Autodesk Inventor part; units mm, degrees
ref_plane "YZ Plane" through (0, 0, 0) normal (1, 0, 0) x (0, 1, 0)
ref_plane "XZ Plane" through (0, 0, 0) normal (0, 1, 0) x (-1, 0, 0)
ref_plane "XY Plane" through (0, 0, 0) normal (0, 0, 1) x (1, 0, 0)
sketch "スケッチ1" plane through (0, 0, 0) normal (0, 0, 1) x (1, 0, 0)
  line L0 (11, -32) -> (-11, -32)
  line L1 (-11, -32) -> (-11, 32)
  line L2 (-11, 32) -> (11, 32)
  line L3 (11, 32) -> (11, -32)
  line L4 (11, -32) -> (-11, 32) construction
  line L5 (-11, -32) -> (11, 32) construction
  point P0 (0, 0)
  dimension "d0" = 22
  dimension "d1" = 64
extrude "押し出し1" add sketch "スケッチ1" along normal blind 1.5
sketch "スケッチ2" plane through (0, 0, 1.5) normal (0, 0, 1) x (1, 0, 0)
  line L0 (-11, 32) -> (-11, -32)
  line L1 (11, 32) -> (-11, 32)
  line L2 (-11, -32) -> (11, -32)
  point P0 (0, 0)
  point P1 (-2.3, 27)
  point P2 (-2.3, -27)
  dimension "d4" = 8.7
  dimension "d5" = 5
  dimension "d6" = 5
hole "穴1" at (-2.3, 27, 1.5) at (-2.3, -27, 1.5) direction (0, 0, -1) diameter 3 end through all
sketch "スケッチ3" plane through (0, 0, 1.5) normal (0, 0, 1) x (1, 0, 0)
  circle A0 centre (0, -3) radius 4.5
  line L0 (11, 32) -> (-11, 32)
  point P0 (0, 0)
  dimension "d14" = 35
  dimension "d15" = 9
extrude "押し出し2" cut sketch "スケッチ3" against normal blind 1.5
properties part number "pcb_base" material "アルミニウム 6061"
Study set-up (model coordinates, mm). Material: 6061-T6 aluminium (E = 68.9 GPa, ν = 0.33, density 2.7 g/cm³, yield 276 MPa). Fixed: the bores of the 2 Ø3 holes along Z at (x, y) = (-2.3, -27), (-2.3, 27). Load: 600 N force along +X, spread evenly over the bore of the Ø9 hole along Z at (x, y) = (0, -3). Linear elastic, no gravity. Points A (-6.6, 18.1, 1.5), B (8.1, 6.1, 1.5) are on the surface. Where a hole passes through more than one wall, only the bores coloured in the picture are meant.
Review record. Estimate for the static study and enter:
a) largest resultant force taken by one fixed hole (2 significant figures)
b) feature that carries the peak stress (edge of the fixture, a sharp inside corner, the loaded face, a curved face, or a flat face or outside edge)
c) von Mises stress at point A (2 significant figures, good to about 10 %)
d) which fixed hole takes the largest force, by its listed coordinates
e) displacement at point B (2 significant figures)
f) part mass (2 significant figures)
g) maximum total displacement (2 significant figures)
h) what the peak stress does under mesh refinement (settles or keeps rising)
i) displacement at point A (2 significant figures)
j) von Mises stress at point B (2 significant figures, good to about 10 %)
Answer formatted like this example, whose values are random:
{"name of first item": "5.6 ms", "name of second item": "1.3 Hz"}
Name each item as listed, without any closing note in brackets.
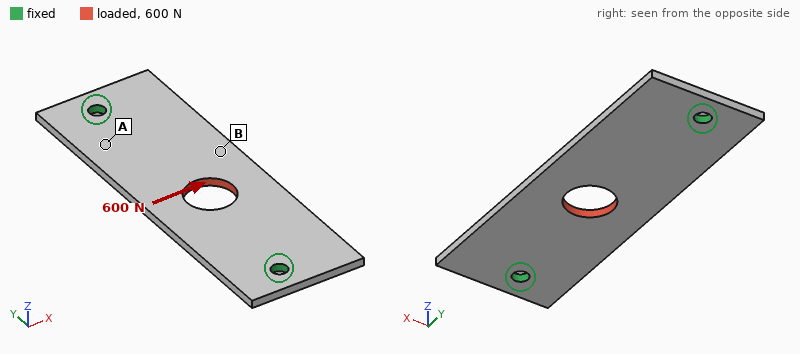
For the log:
{"largest resultant force taken by one fixed hole": "350 N", "feature that carries the peak stress": "edge of the fixture", "von Mises stress at point A": "13 MPa", "which fixed hole takes the largest force, by its listed coordinates": "(-2.3, -27)", "displacement at point B": "23 µm", "part mass": "5.4 g", "maximum total displacement": "27 µm", "what the peak stress does under mesh refinement": "keeps rising", "displacement at point A": "11 µm", "von Mises stress at point B": "33 MPa"}
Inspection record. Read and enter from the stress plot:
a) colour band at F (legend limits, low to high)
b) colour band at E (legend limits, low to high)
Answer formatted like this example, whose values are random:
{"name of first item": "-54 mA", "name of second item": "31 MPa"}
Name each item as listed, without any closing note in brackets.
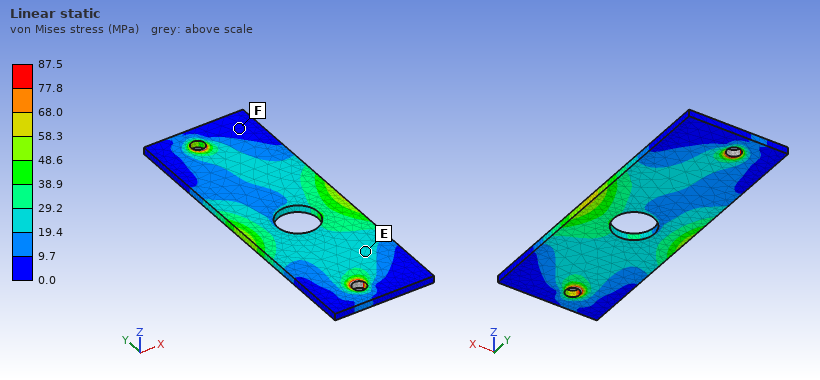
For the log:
{"colour band at F": "0.0 to 9.7 MPa", "colour band at E": "19.4 to 29.2 MPa"}
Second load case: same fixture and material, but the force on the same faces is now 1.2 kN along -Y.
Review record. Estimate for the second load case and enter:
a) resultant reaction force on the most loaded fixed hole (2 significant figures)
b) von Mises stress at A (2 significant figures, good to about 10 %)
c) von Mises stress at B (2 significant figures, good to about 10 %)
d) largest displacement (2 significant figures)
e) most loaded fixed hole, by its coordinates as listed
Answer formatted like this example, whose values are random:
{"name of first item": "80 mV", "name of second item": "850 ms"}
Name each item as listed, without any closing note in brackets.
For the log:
{"resultant reaction force on the most loaded fixed hole": "640 N", "von Mises stress at A": "21 MPa", "von Mises stress at B": "12 MPa", "largest displacement": "11 µm", "most loaded fixed hole, by its coordinates as listed": "(-2.3, -27)"}
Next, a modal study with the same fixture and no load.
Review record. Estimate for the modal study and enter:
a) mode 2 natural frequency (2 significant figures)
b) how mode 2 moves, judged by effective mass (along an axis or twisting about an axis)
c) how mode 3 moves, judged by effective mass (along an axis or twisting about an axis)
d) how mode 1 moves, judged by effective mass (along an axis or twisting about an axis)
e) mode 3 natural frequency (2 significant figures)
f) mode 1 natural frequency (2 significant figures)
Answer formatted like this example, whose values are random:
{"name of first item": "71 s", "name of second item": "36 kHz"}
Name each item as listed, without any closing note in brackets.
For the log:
{"mode 2 natural frequency": "3800 Hz", "how mode 2 moves, judged by effective mass": "twisting about Y", "how mode 3 moves, judged by effective mass": "twisting about X", "how mode 1 moves, judged by effective mass": "along Z", "mode 3 natural frequency": "6100 Hz", "mode 1 natural frequency": "2500 Hz"}
